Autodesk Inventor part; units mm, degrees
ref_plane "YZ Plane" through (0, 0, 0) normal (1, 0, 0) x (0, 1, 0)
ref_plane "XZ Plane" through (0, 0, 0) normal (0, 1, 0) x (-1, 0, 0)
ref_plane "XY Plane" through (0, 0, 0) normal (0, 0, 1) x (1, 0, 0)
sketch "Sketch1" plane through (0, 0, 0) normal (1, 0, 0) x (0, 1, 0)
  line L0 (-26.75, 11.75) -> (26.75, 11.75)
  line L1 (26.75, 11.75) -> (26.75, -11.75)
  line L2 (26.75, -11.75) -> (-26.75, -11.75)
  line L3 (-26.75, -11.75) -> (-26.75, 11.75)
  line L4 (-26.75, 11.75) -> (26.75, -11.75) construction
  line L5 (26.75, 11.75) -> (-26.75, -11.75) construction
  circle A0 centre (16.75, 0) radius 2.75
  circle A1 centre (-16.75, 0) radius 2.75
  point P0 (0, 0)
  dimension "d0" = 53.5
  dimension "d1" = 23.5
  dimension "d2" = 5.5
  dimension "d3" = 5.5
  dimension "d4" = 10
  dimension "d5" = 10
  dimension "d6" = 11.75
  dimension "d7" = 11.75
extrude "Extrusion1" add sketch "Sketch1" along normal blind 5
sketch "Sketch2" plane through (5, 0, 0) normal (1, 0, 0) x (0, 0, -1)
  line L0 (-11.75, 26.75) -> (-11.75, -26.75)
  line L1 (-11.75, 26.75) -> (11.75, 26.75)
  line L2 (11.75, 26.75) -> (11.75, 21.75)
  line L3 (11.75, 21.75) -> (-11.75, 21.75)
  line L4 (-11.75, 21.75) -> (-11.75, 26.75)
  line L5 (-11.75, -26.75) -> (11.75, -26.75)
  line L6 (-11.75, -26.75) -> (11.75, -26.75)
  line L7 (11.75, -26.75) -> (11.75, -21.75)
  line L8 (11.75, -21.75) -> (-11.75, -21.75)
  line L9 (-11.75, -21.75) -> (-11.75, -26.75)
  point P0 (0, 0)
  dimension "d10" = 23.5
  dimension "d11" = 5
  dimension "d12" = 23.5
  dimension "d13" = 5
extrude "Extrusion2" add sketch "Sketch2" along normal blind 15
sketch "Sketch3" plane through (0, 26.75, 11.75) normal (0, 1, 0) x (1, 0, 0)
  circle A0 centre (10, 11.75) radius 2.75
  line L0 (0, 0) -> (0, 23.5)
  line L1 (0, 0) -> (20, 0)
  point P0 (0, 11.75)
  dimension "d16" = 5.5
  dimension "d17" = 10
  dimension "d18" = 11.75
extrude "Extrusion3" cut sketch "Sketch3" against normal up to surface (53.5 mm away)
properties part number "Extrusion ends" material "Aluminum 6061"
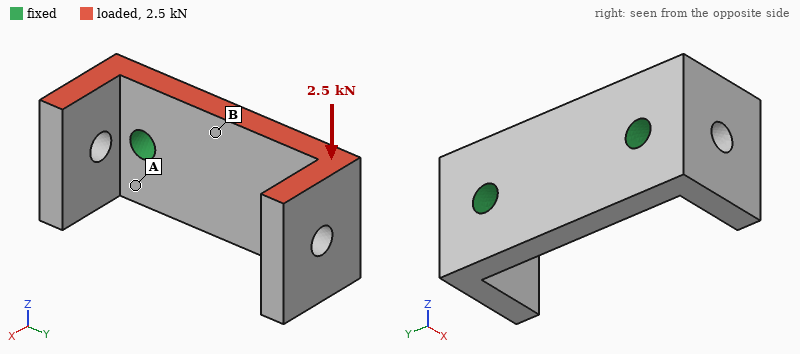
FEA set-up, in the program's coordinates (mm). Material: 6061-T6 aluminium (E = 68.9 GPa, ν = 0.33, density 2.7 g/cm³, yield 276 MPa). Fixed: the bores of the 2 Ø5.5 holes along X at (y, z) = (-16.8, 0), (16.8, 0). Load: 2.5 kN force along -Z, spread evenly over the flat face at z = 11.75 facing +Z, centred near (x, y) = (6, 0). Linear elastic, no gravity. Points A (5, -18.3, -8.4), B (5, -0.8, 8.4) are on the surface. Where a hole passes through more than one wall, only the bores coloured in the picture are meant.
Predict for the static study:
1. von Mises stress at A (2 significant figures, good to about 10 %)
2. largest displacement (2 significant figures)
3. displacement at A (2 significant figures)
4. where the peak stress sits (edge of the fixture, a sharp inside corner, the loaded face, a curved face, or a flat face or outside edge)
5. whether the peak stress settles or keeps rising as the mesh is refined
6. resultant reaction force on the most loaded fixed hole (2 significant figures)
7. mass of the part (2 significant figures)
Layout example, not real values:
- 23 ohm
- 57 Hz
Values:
- 18 MPa
- 26 µm
- 5.2 µm
- edge of the fixture
- keeps rising
- 1.3 kN
- 25 g
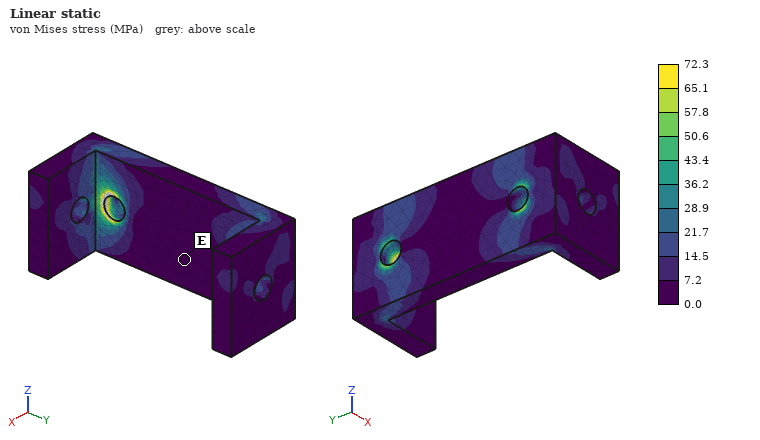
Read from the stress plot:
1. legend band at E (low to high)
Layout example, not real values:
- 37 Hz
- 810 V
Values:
- 0.0 to 7.2 MPa
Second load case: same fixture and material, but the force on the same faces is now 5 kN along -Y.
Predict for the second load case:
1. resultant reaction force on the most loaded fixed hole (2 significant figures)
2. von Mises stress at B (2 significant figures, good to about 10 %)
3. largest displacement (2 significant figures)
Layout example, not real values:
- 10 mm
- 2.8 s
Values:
- 2.8 kN
- 19 MPa
- 0.17 mm
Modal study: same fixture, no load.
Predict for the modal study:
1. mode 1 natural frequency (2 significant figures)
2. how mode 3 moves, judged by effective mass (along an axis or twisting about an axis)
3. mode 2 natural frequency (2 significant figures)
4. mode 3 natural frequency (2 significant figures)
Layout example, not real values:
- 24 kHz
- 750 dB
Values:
- 8300 Hz
- along Z
- 8300 Hz
- 11 kHz
